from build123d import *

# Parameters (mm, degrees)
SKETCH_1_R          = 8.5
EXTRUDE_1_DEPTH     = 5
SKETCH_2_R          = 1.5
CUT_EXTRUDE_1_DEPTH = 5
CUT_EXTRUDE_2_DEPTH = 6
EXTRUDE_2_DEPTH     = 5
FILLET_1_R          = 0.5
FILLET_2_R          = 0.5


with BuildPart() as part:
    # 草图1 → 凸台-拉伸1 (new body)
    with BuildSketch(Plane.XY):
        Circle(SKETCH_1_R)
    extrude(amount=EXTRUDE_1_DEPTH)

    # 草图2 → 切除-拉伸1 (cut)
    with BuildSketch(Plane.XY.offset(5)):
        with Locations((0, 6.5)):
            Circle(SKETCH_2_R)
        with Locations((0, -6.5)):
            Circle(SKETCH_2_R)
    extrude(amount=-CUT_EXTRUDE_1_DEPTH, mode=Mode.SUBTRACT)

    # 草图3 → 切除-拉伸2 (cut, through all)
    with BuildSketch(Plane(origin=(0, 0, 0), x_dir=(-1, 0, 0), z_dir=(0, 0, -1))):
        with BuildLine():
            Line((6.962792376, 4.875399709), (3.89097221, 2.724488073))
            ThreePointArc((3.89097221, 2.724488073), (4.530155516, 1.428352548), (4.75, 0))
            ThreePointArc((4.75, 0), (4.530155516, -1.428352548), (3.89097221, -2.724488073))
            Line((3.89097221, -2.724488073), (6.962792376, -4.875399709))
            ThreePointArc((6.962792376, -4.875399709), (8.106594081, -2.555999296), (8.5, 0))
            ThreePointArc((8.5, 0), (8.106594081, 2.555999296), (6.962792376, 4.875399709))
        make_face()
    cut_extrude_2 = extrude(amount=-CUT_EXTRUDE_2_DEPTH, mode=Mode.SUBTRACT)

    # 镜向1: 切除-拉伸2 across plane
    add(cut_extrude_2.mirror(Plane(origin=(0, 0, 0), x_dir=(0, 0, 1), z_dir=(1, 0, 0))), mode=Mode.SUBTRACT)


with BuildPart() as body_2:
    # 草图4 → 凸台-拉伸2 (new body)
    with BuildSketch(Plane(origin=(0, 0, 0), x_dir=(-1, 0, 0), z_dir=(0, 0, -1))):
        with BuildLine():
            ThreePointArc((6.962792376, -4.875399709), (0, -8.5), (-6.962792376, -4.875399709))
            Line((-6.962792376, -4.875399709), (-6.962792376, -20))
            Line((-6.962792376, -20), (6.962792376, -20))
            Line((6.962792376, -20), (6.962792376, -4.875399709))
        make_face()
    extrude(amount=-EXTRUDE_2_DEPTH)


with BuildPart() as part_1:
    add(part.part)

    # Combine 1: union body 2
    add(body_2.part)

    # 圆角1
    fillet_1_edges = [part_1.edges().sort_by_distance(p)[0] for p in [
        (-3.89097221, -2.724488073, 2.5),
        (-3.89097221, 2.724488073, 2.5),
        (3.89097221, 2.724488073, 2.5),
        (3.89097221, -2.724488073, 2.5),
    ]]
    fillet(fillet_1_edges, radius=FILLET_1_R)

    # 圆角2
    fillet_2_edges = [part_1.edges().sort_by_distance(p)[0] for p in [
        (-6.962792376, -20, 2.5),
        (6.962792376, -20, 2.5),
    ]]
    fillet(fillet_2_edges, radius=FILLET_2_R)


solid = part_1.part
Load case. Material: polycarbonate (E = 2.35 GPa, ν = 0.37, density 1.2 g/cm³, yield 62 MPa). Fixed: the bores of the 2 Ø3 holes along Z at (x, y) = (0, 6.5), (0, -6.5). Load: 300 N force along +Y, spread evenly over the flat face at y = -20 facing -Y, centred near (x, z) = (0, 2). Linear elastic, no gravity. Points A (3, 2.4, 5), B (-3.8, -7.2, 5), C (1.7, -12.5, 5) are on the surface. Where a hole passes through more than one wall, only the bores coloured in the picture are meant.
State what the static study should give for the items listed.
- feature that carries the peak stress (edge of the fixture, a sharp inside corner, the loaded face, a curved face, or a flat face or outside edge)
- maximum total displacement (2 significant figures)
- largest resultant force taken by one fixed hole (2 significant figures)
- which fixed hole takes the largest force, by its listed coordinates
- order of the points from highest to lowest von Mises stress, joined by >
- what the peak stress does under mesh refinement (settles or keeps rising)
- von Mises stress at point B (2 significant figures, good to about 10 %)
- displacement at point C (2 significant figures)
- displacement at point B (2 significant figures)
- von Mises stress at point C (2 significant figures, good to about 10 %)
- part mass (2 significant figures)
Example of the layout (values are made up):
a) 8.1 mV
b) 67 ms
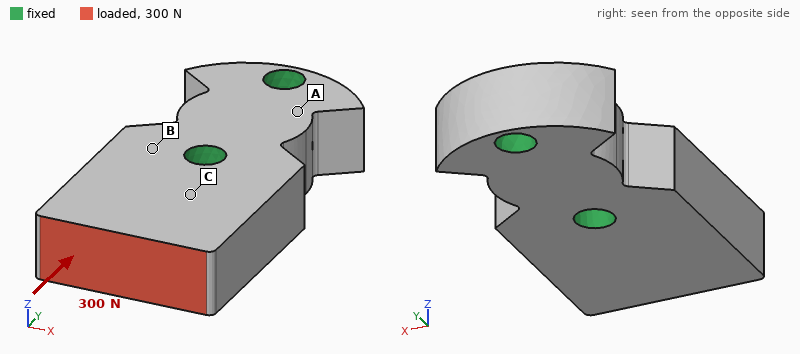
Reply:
a) edge of the fixture
b) 31 µm
c) 270 N
d) (0, -6.5)
e) C > B > A
f) keeps rising
g) 3.0 MPa
h) 15 µm
i) 8.9 µm
j) 5.8 MPa
k) 2.0 g
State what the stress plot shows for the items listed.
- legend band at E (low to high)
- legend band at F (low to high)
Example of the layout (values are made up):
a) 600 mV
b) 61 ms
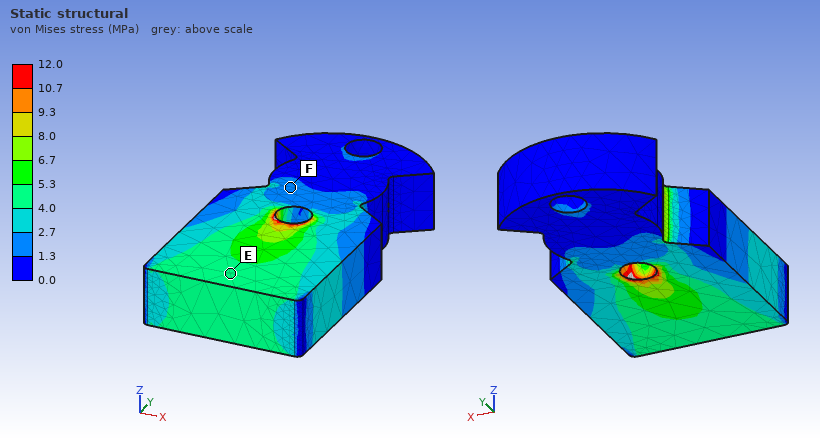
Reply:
a) 4.0 to 5.3 MPa
b) 1.3 to 2.7 MPa
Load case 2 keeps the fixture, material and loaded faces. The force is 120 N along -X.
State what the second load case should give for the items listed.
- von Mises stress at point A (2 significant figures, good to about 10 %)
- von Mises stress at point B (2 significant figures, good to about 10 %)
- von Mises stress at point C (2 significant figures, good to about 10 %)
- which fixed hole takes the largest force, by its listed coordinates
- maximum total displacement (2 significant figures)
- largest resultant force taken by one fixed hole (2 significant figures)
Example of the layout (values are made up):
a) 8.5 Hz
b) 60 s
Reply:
a) 3.3 MPa
b) 7.9 MPa
c) 4.5 MPa
d) (0, -6.5)
e) 0.17 mm
f) 190 N
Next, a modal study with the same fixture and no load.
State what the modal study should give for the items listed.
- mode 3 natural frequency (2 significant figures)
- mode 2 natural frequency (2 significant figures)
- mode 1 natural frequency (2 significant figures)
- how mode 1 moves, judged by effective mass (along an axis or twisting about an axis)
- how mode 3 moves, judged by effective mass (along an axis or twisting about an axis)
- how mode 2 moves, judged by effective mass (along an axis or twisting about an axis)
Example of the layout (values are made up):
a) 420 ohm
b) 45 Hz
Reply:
a) 9100 Hz
b) 6800 Hz
c) 5400 Hz
d) along Z
e) twisting about Y
f) along X
